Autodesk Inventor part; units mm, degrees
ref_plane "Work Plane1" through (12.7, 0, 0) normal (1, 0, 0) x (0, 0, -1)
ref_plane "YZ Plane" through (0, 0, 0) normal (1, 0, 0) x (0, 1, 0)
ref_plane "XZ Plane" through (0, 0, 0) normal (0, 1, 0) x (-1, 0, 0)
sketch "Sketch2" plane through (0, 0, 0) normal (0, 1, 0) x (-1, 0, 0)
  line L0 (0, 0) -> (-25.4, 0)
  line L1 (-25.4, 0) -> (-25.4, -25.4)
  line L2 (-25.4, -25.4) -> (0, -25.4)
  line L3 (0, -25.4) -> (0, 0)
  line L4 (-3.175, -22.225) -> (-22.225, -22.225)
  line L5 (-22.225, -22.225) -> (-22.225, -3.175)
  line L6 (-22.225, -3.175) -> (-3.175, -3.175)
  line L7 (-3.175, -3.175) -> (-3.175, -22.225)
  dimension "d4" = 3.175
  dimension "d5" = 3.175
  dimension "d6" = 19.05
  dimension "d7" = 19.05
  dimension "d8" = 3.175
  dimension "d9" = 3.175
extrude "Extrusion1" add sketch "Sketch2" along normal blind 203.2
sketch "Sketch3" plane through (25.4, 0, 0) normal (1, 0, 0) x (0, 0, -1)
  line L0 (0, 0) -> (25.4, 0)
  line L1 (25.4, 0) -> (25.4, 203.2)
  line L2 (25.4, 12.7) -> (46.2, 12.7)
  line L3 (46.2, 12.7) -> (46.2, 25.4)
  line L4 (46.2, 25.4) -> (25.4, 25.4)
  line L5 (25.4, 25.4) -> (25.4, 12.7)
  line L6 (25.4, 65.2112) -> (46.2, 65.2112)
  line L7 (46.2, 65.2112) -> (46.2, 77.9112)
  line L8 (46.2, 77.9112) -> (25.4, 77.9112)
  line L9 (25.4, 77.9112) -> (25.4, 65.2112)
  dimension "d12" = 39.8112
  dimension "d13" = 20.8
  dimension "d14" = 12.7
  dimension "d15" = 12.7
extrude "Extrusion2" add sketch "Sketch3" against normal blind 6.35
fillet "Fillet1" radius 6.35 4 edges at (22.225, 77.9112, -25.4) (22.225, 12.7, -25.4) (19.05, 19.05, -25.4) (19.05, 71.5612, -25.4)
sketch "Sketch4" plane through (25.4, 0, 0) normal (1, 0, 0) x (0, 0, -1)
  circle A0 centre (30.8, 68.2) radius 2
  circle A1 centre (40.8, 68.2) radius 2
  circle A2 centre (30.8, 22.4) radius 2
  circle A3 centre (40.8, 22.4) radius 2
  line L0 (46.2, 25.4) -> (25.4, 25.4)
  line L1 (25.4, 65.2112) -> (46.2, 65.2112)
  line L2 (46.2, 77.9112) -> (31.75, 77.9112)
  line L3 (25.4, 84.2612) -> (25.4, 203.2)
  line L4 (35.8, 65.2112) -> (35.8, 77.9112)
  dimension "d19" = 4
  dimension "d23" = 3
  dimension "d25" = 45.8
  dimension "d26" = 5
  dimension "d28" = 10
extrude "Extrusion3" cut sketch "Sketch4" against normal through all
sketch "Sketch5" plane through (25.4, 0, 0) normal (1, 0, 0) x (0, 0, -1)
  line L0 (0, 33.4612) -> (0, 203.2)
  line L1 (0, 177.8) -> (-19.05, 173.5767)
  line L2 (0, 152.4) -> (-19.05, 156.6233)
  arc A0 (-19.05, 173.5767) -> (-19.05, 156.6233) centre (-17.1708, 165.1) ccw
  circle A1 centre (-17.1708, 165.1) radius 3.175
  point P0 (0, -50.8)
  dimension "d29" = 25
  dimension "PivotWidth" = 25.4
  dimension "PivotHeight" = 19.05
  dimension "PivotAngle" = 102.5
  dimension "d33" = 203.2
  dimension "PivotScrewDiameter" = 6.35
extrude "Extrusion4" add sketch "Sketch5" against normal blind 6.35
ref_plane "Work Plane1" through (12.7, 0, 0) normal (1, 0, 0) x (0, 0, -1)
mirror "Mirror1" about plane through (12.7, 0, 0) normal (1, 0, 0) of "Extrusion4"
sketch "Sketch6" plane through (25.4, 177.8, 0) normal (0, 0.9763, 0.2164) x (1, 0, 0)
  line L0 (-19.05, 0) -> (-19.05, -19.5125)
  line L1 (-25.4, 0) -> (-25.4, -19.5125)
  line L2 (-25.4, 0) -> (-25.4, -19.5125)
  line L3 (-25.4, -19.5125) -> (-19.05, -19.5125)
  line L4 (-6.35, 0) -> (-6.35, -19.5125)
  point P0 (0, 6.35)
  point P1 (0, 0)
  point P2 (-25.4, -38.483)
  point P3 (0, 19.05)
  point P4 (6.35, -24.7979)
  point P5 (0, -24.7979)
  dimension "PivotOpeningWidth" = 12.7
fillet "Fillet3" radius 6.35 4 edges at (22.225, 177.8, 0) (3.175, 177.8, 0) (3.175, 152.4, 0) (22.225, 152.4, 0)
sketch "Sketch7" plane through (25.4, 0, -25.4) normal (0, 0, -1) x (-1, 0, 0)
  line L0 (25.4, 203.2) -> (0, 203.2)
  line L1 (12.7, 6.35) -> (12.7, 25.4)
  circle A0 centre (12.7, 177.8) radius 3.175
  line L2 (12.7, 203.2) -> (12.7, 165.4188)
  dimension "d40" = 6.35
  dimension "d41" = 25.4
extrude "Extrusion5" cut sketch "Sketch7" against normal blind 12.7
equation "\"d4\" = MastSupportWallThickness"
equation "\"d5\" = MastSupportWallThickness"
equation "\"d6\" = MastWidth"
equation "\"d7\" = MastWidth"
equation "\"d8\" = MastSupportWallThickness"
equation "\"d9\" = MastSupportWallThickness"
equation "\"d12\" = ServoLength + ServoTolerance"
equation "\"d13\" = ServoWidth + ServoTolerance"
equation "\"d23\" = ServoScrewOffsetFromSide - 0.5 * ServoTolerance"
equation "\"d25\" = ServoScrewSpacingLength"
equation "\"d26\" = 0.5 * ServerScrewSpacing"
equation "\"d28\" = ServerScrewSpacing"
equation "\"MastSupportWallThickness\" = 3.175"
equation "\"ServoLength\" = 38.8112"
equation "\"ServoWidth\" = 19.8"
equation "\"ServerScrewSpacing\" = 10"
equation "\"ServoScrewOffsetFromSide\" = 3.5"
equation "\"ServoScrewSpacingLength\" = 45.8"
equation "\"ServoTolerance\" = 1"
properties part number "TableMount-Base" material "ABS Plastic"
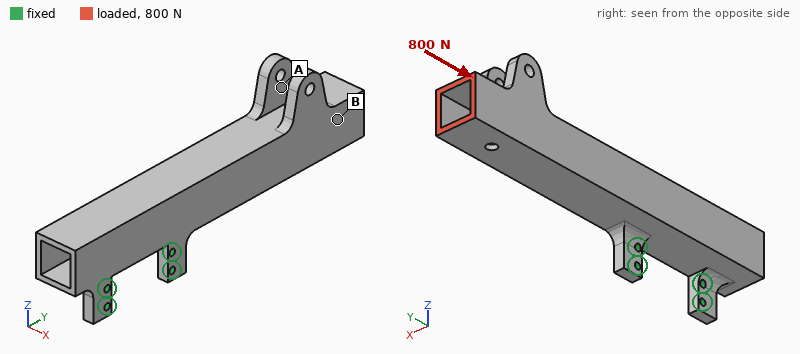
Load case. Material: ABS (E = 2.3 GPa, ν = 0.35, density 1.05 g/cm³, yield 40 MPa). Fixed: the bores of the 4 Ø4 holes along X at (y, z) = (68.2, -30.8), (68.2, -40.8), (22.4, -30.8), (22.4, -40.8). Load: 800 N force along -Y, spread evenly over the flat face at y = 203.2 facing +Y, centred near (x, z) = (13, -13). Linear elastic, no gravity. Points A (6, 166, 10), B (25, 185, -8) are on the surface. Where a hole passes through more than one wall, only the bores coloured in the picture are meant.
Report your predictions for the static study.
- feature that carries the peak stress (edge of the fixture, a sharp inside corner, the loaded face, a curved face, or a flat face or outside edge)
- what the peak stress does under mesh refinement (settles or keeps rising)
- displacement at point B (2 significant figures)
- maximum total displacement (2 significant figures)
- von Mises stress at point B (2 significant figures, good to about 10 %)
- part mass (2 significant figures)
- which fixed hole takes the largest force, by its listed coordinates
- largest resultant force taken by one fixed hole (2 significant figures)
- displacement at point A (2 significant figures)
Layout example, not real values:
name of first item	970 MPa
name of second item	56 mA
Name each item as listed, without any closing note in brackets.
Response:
feature that carries the peak stress	edge of the fixture
what the peak stress does under mesh refinement	keeps rising
displacement at point B	0.75 mm
maximum total displacement	0.90 mm
von Mises stress at point B	2.6 MPa
part mass	70 g
which fixed hole takes the largest force, by its listed coordinates	(68.2, -30.8)
largest resultant force taken by one fixed hole	590 N
displacement at point A	0.72 mm
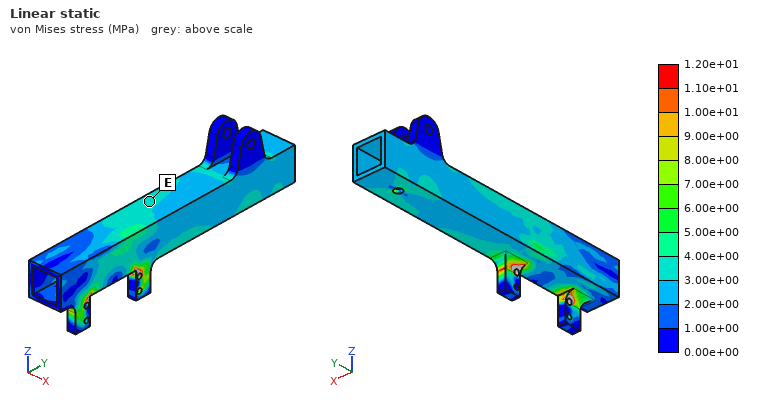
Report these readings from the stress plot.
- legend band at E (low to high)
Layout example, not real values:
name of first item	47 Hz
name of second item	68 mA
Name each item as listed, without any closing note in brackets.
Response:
legend band at E	3.00e+00 to 4.00e+00 MPa
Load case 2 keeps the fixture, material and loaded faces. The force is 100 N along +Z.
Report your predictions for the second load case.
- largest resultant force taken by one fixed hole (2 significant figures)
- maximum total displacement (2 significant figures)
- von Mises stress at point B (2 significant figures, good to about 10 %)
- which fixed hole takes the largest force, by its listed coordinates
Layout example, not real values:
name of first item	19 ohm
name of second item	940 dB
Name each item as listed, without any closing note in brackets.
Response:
largest resultant force taken by one fixed hole	270 N
maximum total displacement	2.6 mm
von Mises stress at point B	1.4 MPa
which fixed hole takes the largest force, by its listed coordinates	(22.4, -30.8)
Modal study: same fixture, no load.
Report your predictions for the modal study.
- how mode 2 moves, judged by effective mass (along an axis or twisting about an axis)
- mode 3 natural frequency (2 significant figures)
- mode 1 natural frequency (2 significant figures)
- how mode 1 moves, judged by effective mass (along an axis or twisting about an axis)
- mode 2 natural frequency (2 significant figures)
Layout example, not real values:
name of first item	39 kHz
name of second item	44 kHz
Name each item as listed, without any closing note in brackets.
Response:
how mode 2 moves, judged by effective mass	along Z
mode 3 natural frequency	450 Hz
mode 1 natural frequency	210 Hz
how mode 1 moves, judged by effective mass	along X
mode 2 natural frequency	270 Hz
